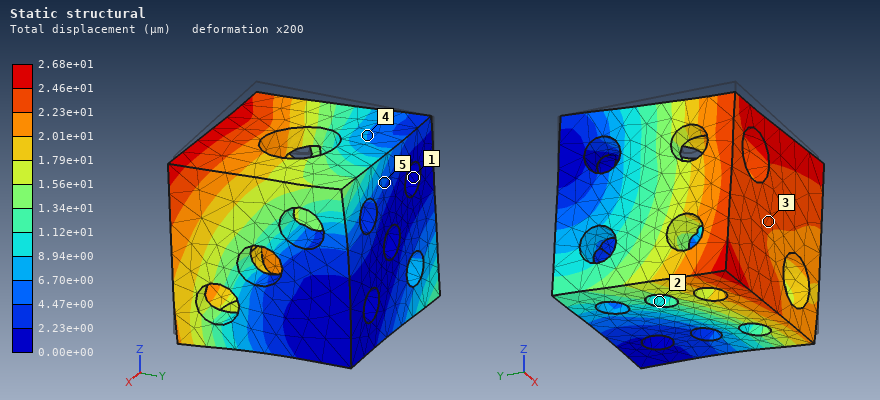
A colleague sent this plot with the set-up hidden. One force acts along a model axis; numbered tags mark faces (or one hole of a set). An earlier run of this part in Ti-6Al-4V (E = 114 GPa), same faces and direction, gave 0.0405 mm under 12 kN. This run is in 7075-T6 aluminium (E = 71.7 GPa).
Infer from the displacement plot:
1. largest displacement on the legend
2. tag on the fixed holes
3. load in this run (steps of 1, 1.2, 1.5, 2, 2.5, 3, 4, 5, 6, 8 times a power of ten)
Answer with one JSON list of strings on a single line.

["2.68e+01 µm", "1", "5 kN"]
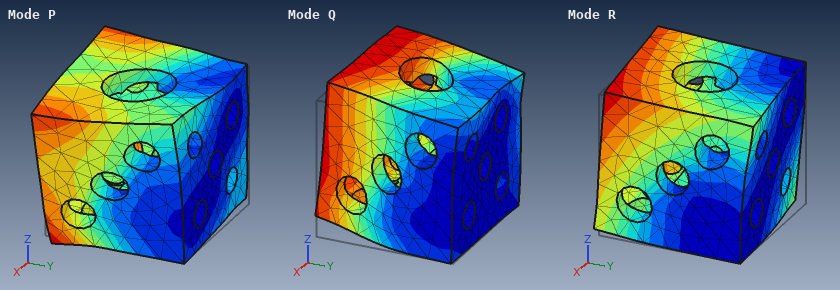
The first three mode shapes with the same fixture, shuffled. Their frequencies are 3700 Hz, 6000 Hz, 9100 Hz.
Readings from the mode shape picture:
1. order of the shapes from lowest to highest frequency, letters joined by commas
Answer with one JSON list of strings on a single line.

["R, Q, P"]
